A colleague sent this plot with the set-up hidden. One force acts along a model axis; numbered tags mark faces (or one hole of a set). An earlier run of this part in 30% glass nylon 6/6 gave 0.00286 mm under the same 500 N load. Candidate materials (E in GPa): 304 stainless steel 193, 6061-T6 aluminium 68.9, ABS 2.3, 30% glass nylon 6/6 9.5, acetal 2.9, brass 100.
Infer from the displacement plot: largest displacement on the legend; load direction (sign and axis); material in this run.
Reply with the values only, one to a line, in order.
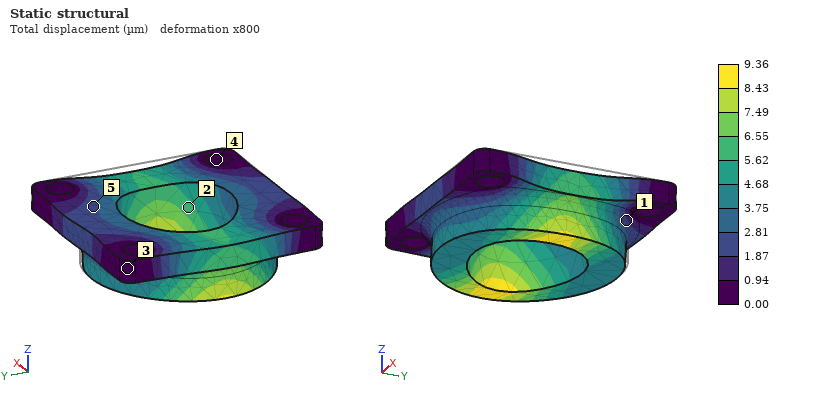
9.36 µm
-X
acetal
